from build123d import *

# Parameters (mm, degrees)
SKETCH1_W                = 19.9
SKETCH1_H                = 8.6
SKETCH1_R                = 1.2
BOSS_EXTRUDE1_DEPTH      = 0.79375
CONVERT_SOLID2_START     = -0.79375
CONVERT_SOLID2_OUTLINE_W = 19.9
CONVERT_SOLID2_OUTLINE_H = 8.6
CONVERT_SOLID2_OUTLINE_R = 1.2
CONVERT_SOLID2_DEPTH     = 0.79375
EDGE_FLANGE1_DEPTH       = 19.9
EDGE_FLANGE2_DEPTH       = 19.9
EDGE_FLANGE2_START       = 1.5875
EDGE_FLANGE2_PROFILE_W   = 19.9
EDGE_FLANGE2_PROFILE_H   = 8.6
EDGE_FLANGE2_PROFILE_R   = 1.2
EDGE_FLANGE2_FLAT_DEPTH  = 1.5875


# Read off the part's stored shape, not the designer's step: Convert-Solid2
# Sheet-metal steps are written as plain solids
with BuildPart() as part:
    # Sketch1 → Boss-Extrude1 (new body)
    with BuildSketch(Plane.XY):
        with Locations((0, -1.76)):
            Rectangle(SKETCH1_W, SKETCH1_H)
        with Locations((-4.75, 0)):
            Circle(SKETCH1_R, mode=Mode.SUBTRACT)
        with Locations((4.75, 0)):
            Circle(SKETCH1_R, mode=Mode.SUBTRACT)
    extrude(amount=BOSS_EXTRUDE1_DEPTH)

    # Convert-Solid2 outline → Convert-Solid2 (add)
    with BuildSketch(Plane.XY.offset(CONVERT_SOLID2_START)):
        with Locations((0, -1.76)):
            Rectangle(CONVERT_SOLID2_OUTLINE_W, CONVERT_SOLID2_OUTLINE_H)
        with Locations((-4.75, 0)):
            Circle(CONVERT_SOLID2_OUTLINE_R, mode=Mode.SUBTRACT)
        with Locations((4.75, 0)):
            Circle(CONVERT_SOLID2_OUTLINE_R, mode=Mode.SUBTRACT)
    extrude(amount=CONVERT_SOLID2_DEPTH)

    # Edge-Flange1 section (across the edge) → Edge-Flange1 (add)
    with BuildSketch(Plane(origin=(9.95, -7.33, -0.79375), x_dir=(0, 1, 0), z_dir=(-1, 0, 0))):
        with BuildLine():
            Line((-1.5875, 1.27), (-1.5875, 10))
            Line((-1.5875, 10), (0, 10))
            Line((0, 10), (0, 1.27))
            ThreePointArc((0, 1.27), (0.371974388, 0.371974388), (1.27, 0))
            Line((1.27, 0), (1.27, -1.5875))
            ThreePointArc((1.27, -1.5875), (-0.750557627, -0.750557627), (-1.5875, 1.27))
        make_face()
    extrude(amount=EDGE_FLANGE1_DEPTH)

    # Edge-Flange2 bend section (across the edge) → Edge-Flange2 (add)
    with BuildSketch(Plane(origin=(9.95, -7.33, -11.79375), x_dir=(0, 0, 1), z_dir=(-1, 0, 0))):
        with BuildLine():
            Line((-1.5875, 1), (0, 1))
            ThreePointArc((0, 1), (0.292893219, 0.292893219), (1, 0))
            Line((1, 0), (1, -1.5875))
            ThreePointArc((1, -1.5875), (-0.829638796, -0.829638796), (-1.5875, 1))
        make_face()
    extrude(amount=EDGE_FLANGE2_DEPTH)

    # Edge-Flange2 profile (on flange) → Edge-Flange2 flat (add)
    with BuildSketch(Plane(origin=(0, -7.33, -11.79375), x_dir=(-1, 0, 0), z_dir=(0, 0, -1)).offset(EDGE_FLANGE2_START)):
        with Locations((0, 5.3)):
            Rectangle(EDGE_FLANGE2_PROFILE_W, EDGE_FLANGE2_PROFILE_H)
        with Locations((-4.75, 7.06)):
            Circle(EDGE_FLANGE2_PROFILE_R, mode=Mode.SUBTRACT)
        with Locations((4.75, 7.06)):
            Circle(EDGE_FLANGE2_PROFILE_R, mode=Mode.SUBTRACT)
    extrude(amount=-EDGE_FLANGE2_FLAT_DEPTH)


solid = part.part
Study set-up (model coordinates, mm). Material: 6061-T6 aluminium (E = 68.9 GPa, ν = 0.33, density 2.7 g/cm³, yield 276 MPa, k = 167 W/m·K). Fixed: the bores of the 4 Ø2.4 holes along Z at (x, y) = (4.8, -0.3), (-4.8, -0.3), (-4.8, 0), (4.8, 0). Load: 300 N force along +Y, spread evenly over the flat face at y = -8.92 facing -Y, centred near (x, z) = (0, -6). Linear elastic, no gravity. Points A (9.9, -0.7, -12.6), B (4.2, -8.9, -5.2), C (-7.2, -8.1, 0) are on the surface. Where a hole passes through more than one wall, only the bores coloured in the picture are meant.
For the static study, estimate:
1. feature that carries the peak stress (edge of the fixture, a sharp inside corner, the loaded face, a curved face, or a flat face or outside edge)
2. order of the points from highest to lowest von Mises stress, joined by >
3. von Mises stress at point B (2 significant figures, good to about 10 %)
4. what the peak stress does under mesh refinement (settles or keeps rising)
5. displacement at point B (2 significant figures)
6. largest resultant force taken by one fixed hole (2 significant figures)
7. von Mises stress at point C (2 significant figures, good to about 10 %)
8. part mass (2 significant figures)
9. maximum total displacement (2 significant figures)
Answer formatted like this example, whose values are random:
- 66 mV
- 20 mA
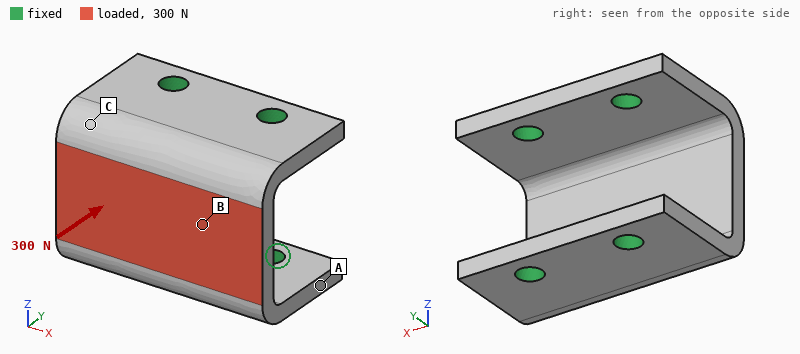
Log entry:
- edge of the fixture
- B > C > A
- 27 MPa
- keeps rising
- 7.1 µm
- 83 N
- 15 MPa
- 2.7 g
- 9.0 µm
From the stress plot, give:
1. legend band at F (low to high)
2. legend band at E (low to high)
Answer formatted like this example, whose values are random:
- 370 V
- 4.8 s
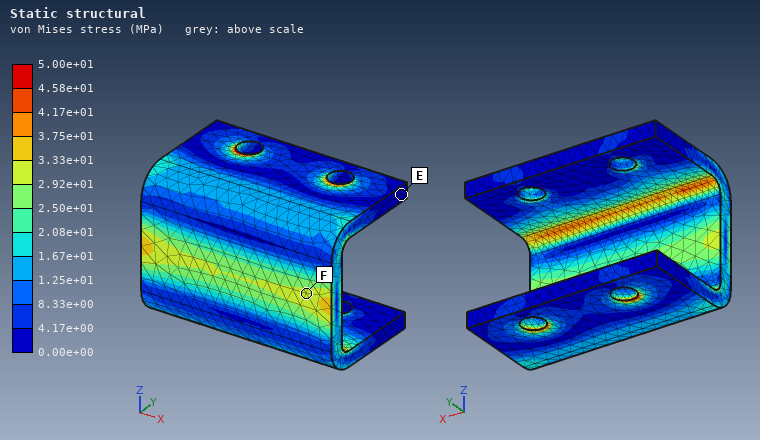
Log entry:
- 2.92e+01 to 3.33e+01 MPa
- 0.00e+00 to 4.17e+00 MPa
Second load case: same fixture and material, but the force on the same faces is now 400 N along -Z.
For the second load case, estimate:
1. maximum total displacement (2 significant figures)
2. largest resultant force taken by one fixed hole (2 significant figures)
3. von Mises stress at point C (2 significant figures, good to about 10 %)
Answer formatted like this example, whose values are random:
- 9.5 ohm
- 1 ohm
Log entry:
- 24 µm
- 120 N
- 34 MPa
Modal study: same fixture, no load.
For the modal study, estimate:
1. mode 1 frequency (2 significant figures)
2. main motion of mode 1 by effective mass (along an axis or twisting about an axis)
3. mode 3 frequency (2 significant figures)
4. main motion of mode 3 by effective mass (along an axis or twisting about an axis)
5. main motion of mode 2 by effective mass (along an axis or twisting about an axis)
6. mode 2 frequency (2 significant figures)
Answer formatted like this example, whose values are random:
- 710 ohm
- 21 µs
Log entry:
- 17 kHz
- along Z
- 37 kHz
- twisting about Y
- along X
- 36 kHz
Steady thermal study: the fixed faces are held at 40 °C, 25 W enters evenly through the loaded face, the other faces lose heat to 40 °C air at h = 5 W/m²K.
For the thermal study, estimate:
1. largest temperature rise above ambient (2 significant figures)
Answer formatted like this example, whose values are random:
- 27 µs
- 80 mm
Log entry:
- 27 K
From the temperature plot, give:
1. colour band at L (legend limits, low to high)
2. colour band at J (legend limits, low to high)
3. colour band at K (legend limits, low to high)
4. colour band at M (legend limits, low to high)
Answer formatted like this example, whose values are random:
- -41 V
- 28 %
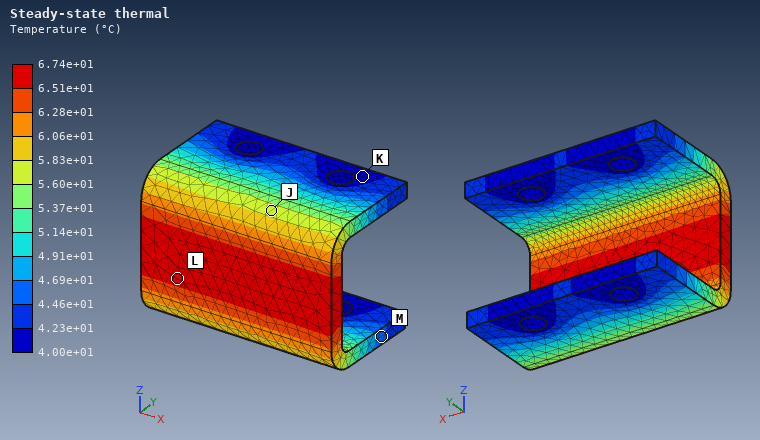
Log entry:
- 6.51e+01 to 6.74e+01 °C
- 5.60e+01 to 5.83e+01 °C
- 4.00e+01 to 4.23e+01 °C
- 4.46e+01 to 4.69e+01 °C
